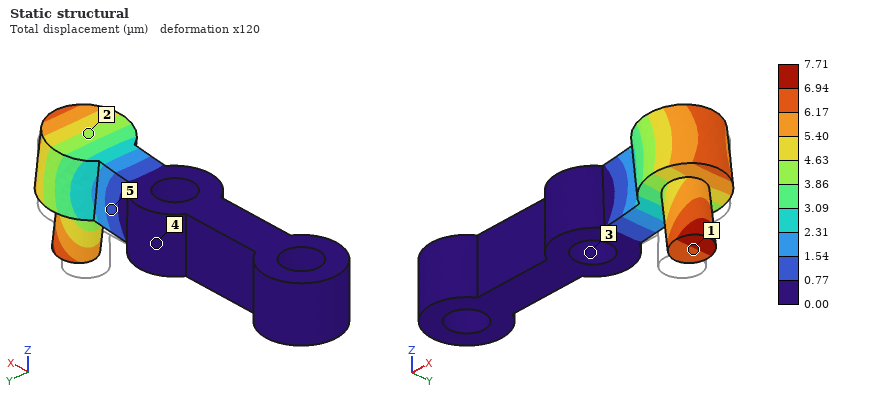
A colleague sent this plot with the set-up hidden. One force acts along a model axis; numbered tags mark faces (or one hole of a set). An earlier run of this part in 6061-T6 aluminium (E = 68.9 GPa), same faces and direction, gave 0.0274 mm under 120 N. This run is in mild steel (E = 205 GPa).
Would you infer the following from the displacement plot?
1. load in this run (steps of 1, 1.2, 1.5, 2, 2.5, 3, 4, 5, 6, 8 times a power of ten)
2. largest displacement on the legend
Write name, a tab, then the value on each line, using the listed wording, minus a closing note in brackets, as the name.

load in this run	100 N
largest displacement on the legend	7.71 µm
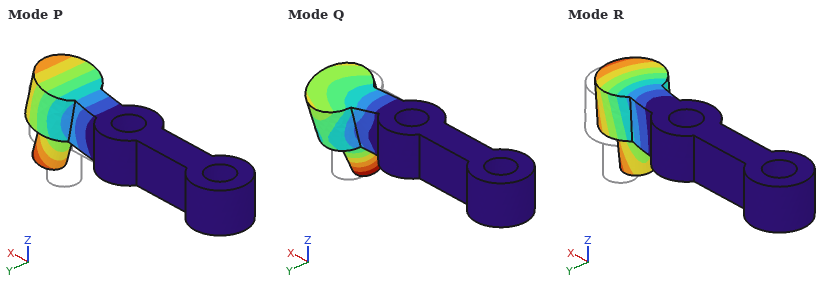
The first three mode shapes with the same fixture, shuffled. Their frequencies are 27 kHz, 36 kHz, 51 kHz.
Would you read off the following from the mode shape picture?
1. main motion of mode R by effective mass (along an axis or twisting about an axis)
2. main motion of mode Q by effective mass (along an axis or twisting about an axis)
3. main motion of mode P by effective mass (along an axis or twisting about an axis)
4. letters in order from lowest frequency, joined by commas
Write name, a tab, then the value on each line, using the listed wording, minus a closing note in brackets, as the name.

main motion of mode R by effective mass	along Y
main motion of mode Q by effective mass	twisting about X
main motion of mode P by effective mass	along Z
letters in order from lowest frequency, joined by commas	R, P, Q
